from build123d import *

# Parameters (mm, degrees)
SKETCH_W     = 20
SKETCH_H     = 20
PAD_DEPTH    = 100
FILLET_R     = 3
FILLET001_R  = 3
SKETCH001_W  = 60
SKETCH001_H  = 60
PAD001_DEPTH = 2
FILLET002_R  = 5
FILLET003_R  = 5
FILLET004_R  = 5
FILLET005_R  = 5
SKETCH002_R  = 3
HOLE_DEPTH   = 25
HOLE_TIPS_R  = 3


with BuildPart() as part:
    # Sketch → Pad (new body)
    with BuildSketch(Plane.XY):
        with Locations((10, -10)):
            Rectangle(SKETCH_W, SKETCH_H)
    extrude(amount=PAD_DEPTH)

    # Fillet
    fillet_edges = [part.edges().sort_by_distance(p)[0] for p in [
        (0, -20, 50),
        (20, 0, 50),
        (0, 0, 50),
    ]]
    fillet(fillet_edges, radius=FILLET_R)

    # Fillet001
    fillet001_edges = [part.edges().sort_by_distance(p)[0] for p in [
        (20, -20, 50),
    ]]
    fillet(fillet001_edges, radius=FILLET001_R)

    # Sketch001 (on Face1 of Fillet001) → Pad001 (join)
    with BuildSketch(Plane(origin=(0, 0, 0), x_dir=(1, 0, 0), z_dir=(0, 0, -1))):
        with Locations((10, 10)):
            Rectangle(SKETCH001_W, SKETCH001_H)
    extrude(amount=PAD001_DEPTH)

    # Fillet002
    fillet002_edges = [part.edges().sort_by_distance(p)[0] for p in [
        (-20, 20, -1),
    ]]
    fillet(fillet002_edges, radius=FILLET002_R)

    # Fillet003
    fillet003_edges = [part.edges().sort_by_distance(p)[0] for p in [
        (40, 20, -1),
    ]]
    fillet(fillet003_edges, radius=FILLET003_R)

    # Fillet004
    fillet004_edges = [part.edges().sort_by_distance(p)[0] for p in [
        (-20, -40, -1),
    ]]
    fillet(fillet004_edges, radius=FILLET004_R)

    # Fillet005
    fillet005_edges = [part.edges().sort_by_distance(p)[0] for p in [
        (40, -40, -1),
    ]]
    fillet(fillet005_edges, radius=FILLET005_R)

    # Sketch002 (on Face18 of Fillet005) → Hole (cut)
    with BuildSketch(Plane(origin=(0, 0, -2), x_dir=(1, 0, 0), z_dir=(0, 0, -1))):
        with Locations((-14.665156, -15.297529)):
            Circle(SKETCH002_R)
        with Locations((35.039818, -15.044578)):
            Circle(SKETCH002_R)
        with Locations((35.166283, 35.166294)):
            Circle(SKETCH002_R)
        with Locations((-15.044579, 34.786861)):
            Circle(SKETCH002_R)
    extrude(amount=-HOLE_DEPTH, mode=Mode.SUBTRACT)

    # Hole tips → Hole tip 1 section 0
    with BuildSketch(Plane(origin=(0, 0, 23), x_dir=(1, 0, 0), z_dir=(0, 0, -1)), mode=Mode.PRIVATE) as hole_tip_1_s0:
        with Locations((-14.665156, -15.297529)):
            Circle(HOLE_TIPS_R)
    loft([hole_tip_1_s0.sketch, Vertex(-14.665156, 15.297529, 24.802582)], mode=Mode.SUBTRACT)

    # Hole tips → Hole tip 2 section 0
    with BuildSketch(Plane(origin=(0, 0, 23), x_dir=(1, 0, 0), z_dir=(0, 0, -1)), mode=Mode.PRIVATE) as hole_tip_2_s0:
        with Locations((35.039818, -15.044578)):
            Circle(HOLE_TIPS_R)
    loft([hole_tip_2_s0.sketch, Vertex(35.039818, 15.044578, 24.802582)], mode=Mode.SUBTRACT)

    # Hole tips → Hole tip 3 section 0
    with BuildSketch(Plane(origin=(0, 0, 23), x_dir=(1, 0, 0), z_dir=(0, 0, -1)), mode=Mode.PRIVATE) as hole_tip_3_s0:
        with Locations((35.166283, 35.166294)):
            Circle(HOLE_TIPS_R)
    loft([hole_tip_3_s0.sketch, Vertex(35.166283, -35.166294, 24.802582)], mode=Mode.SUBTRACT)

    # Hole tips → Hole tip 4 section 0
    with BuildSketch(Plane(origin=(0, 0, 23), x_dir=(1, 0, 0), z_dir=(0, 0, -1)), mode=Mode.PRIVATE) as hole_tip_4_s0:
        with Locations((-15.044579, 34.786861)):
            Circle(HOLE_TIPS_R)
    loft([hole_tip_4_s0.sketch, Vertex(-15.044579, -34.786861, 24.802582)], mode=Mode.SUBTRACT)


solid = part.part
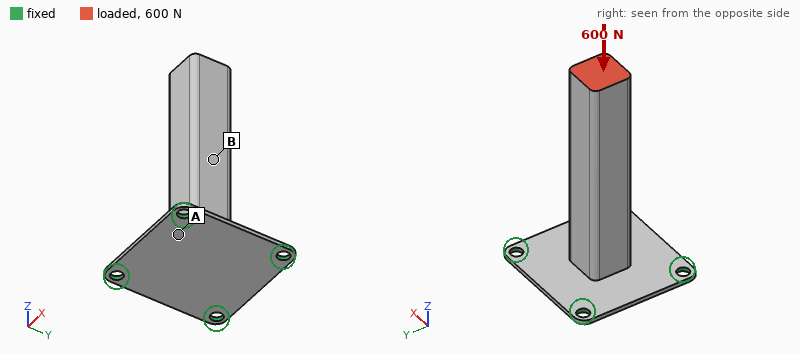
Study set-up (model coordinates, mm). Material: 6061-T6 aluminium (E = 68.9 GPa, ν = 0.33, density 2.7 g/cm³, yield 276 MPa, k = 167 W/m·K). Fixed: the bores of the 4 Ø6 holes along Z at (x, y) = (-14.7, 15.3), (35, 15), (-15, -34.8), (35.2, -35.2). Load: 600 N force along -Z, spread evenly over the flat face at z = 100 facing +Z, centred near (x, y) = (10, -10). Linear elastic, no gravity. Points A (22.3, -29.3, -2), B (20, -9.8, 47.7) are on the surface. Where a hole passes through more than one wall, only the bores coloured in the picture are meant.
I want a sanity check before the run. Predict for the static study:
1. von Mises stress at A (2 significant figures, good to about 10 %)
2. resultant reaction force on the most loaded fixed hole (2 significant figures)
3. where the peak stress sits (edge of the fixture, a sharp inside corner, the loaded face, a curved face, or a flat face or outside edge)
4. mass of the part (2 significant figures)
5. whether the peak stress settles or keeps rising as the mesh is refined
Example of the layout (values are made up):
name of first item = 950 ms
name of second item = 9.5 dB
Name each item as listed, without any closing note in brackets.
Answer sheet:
von Mises stress at A = 22 MPa
resultant reaction force on the most loaded fixed hole = 160 N
where the peak stress sits = edge of the fixture
mass of the part = 120 g
whether the peak stress settles or keeps rising as the mesh is refined = keeps rising
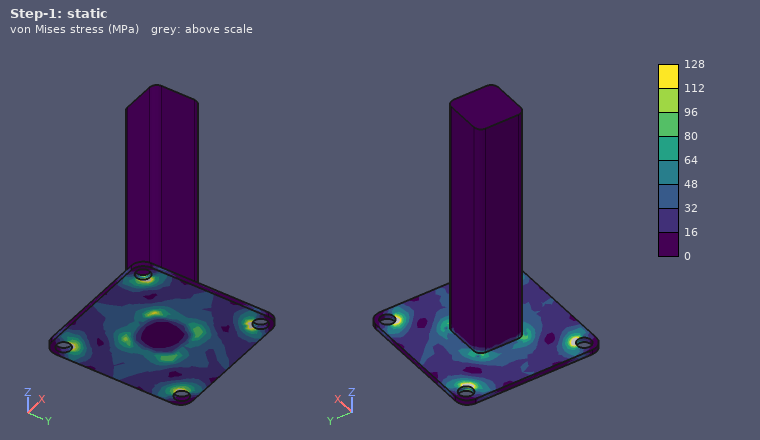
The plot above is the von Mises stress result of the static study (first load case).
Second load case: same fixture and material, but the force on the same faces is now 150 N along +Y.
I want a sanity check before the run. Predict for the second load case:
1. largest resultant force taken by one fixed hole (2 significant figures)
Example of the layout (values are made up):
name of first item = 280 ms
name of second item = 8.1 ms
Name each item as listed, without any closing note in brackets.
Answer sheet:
largest resultant force taken by one fixed hole = 200 N
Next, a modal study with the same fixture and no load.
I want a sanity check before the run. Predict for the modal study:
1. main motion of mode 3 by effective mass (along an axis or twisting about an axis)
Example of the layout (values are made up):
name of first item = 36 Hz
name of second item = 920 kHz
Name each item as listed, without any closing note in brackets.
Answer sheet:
main motion of mode 3 by effective mass = along Z
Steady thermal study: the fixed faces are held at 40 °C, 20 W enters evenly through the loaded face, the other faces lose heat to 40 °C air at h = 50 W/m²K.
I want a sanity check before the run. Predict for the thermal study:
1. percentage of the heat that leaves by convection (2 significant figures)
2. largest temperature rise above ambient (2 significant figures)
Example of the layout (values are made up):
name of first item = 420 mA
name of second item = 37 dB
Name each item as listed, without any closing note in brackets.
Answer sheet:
percentage of the heat that leaves by convection = 47 %
largest temperature rise above ambient = 33 K
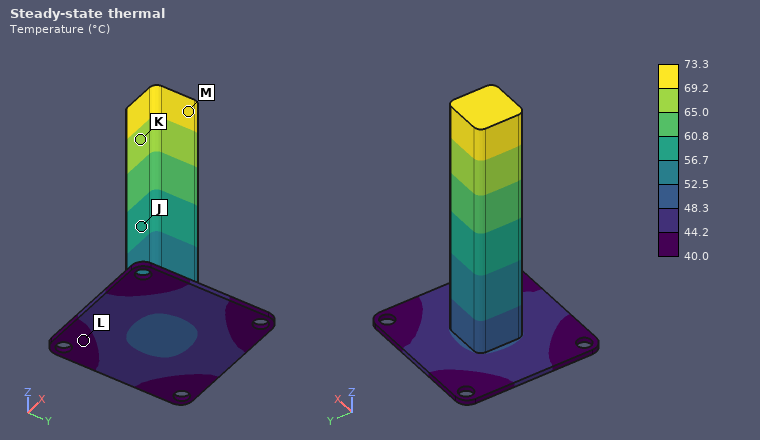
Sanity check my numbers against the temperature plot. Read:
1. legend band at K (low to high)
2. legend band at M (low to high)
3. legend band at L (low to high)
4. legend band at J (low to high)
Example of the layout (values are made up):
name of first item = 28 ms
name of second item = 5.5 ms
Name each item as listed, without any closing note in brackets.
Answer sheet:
legend band at K = 65.0 to 69.2 °C
legend band at M = 69.2 to 73.3 °C
legend band at L = 40.0 to 44.2 °C
legend band at J = 56.7 to 60.8 °C
